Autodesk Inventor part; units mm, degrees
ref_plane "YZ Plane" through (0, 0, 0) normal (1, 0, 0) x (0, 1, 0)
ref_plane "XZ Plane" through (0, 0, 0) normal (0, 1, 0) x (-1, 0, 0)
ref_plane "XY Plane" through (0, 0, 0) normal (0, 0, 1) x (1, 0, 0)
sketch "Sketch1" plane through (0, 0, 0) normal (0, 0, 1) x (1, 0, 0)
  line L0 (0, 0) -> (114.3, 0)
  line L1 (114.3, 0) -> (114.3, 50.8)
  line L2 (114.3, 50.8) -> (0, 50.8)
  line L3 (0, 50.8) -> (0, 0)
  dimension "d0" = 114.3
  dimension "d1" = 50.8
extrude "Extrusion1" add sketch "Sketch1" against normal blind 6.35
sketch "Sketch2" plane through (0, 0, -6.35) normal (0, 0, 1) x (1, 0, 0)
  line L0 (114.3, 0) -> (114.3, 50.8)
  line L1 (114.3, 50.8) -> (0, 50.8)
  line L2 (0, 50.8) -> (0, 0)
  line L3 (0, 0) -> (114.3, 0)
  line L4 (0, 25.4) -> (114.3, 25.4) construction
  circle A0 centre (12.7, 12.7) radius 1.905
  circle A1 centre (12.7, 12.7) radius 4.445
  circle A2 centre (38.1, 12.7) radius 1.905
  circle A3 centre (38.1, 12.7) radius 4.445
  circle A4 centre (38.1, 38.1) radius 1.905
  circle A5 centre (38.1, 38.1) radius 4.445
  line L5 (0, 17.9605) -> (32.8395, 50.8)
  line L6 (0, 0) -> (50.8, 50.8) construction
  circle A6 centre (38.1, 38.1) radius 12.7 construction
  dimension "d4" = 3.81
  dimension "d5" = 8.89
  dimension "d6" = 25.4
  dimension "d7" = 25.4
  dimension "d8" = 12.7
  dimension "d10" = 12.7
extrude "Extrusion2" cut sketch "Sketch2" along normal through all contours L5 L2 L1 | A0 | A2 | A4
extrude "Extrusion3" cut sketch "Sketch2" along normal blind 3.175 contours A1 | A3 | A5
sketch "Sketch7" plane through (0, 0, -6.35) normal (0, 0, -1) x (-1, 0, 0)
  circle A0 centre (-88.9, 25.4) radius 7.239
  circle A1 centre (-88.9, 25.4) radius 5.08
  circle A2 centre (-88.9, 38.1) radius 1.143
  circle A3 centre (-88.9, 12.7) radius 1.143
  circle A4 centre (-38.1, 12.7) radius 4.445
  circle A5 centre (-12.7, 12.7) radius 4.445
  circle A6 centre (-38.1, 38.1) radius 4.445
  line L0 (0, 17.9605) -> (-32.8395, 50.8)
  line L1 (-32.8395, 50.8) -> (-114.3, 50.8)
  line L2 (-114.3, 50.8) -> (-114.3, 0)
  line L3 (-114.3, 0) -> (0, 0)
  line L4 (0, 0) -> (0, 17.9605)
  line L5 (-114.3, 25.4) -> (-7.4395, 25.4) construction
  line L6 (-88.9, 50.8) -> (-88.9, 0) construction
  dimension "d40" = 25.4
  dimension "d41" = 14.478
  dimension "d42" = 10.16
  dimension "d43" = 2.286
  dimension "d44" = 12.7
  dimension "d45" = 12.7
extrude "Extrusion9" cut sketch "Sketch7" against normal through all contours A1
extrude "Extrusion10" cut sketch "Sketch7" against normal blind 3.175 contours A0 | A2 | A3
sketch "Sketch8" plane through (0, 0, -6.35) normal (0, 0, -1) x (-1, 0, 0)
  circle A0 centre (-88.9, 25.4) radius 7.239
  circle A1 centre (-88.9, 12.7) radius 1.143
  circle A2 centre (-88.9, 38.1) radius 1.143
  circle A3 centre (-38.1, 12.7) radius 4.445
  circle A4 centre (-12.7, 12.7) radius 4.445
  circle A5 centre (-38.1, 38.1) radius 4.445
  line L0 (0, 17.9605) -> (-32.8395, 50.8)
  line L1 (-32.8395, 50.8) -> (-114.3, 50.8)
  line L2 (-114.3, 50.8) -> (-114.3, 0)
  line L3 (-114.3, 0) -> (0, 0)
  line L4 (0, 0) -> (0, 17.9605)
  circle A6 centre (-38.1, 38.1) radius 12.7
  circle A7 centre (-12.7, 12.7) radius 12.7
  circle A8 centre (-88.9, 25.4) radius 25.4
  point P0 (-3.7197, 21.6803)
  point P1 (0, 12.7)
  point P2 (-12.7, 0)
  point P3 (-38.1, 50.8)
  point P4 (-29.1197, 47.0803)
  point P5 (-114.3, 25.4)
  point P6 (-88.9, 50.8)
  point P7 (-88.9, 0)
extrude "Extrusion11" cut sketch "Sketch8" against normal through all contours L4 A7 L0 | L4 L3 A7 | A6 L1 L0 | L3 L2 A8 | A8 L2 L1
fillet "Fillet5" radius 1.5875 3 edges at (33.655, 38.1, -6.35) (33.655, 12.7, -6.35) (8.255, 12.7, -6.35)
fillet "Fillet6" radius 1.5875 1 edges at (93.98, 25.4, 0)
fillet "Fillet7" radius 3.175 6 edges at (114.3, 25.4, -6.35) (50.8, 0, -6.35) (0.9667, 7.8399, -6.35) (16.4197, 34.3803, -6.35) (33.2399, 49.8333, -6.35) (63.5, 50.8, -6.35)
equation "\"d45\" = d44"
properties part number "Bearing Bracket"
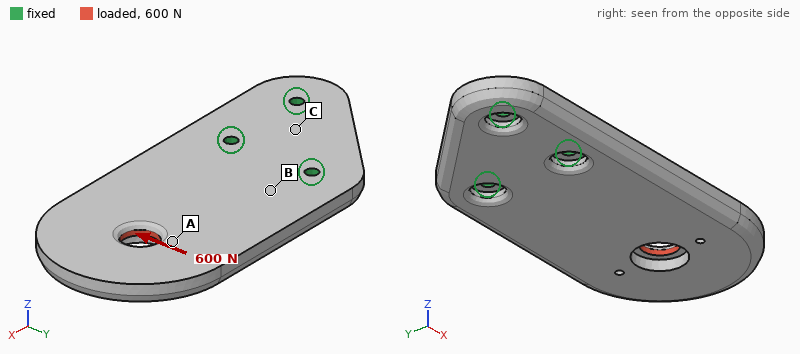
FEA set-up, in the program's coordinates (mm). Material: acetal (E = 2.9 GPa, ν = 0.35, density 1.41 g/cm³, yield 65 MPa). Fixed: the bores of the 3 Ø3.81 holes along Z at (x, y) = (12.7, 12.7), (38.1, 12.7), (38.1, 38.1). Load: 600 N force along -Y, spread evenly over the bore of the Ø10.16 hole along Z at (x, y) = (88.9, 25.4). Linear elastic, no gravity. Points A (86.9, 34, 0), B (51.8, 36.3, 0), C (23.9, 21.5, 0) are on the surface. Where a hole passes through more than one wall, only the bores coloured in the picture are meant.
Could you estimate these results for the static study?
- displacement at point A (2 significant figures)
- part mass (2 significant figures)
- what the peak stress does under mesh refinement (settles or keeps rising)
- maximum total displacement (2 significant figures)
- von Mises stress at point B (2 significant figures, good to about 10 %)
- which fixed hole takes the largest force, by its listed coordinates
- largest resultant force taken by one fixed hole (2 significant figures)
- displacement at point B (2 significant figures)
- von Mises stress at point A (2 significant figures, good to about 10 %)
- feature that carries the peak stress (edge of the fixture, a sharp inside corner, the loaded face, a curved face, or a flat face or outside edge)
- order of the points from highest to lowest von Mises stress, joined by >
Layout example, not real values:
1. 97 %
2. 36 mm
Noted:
1. 0.43 mm
2. 41 g
3. keeps rising
4. 0.64 mm
5. 8.8 MPa
6. (38.1, 38.1)
7. 960 N
8. 0.12 mm
9. 6.1 MPa
10. edge of the fixture
11. B > A > C
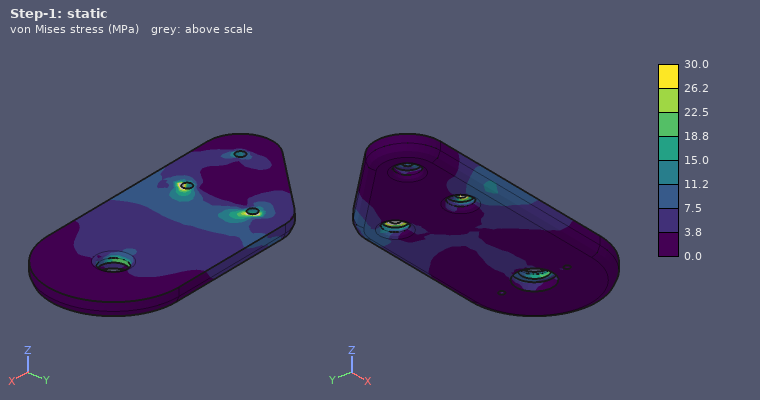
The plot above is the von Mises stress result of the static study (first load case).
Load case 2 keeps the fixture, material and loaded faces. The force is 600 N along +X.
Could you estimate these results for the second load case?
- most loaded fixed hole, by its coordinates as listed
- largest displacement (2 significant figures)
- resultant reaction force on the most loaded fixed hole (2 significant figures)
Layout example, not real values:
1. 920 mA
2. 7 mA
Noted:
1. (38.1, 38.1)
2. 0.25 mm
3. 280 N
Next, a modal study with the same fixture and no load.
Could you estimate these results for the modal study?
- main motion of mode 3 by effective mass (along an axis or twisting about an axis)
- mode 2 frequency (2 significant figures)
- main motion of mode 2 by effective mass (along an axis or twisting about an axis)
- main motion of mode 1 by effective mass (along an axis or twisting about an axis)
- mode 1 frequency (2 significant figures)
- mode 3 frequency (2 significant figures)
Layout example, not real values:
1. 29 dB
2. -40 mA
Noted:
1. along Y
2. 860 Hz
3. twisting about X
4. along Z
5. 250 Hz
6. 1400 Hz
